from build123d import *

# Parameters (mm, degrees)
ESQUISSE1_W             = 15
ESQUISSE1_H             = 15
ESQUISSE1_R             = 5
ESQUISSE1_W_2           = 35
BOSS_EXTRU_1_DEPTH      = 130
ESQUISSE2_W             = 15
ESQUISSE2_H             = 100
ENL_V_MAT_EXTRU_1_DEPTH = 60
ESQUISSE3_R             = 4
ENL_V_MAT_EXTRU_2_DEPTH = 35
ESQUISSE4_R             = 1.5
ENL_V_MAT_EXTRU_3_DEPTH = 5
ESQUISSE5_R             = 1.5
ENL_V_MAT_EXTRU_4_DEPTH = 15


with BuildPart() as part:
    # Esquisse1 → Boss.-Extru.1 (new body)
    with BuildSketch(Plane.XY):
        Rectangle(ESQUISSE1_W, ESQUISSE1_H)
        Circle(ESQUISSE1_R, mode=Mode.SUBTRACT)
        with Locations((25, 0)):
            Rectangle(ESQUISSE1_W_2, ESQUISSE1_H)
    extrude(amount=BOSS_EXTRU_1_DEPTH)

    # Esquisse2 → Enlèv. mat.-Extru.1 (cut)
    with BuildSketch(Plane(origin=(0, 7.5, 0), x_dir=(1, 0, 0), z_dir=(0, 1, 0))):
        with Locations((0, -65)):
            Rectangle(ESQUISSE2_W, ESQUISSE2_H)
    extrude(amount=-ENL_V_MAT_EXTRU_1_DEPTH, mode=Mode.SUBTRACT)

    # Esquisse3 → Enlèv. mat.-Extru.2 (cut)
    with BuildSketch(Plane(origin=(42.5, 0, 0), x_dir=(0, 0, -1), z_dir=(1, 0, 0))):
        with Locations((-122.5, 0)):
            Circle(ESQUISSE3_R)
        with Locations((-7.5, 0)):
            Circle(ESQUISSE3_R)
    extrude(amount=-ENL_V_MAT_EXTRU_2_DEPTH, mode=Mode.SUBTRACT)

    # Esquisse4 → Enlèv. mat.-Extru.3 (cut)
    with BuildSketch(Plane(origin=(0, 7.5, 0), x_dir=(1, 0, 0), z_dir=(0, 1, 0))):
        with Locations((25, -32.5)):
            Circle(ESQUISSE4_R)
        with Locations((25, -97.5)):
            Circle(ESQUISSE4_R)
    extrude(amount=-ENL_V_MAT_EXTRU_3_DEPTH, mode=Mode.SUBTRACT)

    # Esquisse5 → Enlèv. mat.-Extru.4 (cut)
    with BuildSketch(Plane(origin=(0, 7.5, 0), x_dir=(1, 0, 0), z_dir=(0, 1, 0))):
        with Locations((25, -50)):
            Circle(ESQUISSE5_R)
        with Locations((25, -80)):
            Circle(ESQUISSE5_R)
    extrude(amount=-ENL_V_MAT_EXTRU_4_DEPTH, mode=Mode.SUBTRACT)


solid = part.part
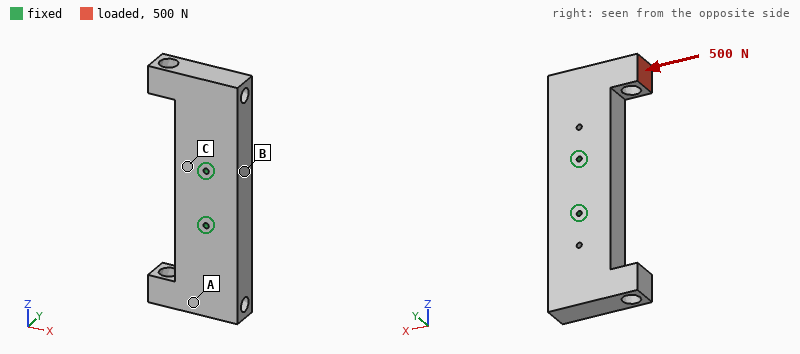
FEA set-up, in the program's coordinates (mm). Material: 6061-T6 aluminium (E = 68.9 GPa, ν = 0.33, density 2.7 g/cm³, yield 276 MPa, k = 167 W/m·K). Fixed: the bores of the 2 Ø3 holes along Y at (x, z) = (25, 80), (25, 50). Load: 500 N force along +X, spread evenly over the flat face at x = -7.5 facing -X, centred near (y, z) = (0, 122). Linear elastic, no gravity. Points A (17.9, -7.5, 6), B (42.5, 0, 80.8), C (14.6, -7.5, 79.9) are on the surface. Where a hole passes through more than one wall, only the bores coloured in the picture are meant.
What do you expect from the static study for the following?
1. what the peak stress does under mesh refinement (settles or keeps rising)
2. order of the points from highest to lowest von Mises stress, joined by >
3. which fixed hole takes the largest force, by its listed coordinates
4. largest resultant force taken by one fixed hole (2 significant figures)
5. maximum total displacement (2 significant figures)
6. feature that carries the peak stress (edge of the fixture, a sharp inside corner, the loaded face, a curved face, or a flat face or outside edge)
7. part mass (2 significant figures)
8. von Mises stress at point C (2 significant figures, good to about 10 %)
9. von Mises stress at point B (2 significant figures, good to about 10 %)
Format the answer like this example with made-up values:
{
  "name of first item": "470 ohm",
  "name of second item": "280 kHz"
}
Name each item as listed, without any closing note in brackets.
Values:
{
  "what the peak stress does under mesh refinement": "keeps rising",
  "order of the points from highest to lowest von Mises stress, joined by >": "B > C > A",
  "which fixed hole takes the largest force, by its listed coordinates": "(25, 80)",
  "largest resultant force taken by one fixed hole": "1.2 kN",
  "maximum total displacement": "19 µm",
  "feature that carries the peak stress": "edge of the fixture",
  "part mass": "190 g",
  "von Mises stress at point C": "4.2 MPa",
  "von Mises stress at point B": "7.2 MPa"
}
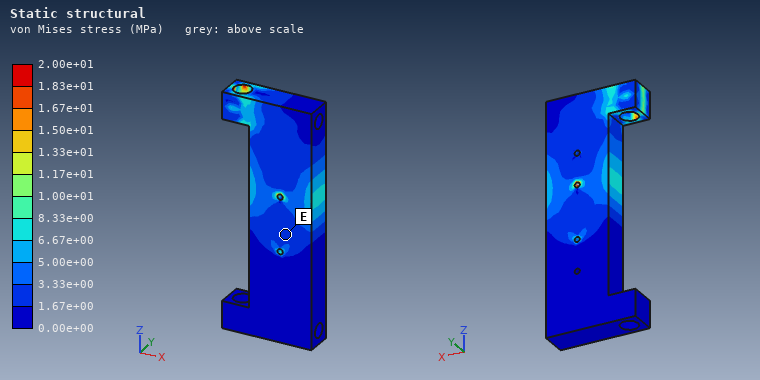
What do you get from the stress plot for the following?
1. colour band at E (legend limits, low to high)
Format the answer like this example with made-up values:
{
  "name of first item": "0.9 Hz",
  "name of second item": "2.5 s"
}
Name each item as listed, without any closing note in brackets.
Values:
{
  "colour band at E": "1.67e+00 to 3.33e+00 MPa"
}
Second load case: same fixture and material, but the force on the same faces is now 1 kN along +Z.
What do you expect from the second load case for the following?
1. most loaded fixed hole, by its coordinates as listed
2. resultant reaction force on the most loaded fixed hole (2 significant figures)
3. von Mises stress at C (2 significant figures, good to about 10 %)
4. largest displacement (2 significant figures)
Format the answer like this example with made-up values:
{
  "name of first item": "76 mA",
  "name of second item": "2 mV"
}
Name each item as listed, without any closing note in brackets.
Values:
{
  "most loaded fixed hole, by its coordinates as listed": "(25, 80)",
  "resultant reaction force on the most loaded fixed hole": "1.2 kN",
  "von Mises stress at C": "7.7 MPa",
  "largest displacement": "59 µm"
}
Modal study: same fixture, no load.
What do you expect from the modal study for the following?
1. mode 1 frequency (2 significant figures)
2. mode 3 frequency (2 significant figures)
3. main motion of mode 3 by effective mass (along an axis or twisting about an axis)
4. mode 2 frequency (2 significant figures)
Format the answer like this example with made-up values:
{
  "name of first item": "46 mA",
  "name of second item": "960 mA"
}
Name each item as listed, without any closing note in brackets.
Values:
{
  "mode 1 frequency": "3700 Hz",
  "mode 3 frequency": "5000 Hz",
  "main motion of mode 3 by effective mass": "twisting about Y",
  "mode 2 frequency": "3700 Hz"
}
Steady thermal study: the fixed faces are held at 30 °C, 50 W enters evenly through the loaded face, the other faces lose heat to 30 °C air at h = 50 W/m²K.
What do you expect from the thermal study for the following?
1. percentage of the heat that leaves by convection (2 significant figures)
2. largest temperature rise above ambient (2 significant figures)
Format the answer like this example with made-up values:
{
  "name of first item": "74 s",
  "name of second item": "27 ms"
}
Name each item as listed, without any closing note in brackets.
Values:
{
  "percentage of the heat that leaves by convection": "18 %",
  "largest temperature rise above ambient": "78 K"
}
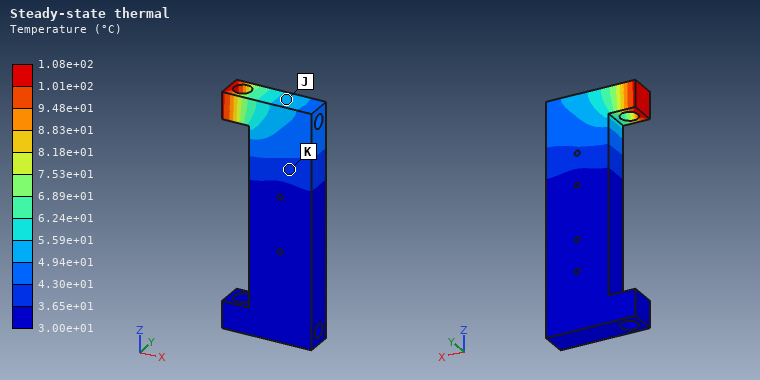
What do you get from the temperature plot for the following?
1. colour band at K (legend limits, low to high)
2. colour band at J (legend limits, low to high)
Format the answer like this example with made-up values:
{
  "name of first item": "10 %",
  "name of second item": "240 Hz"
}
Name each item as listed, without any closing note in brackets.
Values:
{
  "colour band at K": "3.65e+01 to 4.30e+01 °C",
  "colour band at J": "4.94e+01 to 5.59e+01 °C"
}
